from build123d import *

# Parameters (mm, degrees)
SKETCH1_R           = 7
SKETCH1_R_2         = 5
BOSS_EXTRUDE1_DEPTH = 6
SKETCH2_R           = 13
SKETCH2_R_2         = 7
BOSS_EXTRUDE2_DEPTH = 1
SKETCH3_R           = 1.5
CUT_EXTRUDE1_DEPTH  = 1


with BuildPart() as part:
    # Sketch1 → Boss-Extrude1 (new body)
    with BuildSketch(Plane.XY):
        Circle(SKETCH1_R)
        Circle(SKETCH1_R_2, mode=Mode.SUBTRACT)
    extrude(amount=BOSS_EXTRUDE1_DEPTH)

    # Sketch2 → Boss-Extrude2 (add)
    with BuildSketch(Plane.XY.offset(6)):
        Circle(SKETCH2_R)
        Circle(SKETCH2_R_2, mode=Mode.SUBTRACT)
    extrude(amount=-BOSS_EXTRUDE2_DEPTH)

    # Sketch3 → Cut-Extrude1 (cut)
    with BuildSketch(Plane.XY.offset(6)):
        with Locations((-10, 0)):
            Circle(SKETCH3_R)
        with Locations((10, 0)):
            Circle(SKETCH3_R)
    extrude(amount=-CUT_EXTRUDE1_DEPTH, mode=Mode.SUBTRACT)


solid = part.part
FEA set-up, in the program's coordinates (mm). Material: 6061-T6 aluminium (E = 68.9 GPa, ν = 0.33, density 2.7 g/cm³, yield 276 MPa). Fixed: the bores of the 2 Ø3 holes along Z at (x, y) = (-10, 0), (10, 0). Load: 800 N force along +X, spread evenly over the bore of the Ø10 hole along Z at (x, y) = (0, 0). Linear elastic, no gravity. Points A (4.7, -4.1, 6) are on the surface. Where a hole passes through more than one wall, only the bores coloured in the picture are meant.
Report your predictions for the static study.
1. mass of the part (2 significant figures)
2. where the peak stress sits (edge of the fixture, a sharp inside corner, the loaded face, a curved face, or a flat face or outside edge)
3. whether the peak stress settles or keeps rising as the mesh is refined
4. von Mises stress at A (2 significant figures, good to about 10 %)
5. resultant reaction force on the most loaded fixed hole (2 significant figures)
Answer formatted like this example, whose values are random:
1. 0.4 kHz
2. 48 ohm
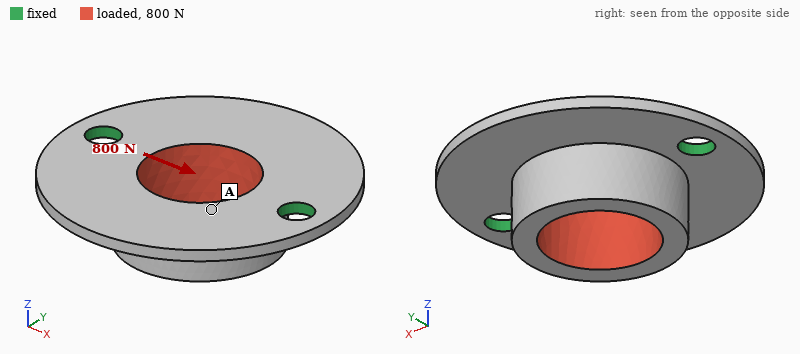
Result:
1. 2.2 g
2. edge of the fixture
3. keeps rising
4. 24 MPa
5. 420 N
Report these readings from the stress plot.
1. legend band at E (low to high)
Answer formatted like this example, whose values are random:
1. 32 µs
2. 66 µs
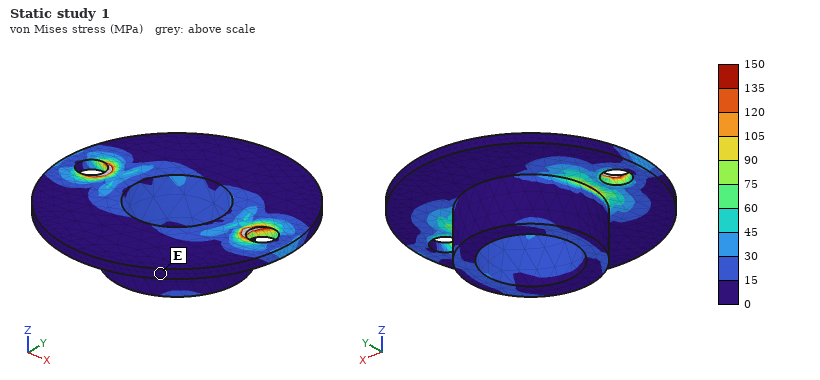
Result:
1. 0 to 15 MPa
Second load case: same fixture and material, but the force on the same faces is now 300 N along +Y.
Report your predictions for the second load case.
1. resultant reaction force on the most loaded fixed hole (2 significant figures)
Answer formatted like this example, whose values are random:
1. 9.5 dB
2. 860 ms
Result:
1. 150 N
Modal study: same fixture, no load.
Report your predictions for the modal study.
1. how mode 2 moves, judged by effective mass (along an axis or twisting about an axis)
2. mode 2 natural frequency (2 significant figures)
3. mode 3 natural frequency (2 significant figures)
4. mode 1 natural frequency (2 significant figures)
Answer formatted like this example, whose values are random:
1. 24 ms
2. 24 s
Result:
1. along Z
2. 13 kHz
3. 20 kHz
4. 6100 Hz
